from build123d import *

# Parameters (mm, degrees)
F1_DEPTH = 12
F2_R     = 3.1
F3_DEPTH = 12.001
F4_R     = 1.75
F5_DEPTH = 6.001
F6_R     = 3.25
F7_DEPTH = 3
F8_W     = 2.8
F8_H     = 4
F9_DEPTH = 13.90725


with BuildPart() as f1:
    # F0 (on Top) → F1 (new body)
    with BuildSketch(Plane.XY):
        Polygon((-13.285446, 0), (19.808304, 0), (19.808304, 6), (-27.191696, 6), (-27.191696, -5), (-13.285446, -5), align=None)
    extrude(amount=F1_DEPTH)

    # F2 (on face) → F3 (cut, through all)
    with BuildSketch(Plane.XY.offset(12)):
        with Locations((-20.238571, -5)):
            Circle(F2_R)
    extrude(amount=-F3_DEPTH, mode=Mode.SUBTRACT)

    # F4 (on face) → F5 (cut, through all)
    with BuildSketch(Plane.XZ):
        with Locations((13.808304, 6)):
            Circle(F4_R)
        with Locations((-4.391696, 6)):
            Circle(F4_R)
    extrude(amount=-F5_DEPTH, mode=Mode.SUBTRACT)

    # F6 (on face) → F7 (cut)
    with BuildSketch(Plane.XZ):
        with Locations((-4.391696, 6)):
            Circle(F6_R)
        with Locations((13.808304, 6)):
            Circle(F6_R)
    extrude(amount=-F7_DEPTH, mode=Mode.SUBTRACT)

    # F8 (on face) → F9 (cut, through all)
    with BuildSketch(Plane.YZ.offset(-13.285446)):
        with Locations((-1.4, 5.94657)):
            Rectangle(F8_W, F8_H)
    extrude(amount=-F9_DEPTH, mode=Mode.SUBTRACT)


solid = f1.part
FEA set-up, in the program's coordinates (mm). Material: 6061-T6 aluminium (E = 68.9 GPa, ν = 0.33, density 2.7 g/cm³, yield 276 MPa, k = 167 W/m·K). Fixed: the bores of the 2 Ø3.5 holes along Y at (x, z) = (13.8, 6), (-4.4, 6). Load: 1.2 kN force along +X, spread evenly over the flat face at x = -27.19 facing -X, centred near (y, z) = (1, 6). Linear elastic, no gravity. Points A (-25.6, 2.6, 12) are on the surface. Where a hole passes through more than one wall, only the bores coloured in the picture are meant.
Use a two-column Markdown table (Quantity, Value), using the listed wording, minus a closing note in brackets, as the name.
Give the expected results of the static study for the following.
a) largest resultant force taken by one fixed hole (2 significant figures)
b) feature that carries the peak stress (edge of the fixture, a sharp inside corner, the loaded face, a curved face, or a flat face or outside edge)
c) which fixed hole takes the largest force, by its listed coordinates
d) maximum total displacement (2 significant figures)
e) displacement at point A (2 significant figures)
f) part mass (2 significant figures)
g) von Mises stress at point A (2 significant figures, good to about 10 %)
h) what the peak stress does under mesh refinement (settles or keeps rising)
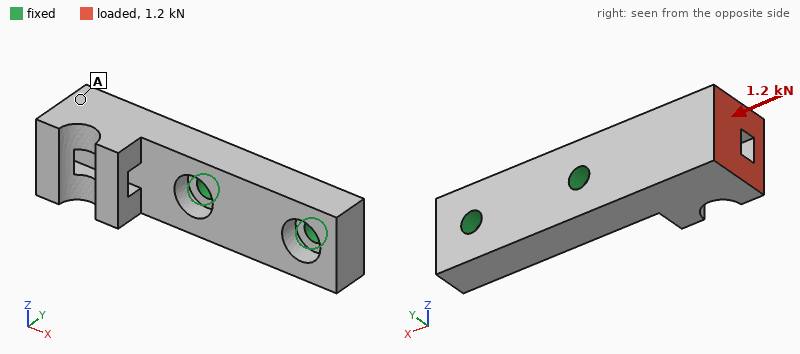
| Quantity | Value |
|---|---|
| largest resultant force taken by one fixed hole | 790 N |
| feature that carries the peak stress | edge of the fixture |
| which fixed hole takes the largest force, by its listed coordinates | (-4.4, 6) |
| maximum total displacement | 87 µm |
| displacement at point A | 68 µm |
| part mass | 9.8 g |
| von Mises stress at point A | 14 MPa |
| what the peak stress does under mesh refinement | keeps rising |
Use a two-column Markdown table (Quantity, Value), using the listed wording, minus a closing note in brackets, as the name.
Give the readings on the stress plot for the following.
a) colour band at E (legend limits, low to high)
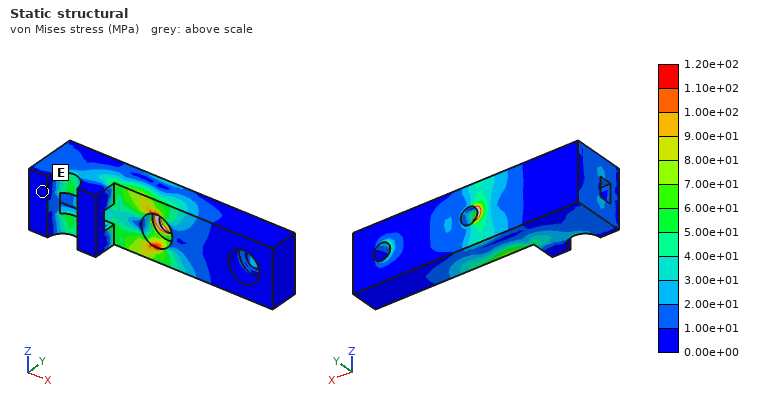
| Quantity | Value |
|---|---|
| colour band at E | 0.00e+00 to 1.00e+01 MPa |
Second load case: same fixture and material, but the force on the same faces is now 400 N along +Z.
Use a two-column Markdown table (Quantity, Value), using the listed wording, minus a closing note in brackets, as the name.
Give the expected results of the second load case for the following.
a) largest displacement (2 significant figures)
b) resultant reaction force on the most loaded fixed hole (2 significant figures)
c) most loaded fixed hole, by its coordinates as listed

| Quantity | Value |
|---|---|
| largest displacement | 67 µm |
| resultant reaction force on the most loaded fixed hole | 730 N |
| most loaded fixed hole, by its coordinates as listed | (-4.4, 6) |
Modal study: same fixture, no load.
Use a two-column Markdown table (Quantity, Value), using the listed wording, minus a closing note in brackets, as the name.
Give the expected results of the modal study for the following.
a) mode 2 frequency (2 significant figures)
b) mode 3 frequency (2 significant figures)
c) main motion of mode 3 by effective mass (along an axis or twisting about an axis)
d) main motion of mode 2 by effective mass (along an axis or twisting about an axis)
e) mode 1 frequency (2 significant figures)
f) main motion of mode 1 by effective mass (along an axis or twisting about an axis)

| Quantity | Value |
|---|---|
| mode 2 frequency | 9000 Hz |
| mode 3 frequency | 15 kHz |
| main motion of mode 3 by effective mass | twisting about X |
| main motion of mode 2 by effective mass | along Z |
| mode 1 frequency | 5600 Hz |
| main motion of mode 1 by effective mass | along Y |
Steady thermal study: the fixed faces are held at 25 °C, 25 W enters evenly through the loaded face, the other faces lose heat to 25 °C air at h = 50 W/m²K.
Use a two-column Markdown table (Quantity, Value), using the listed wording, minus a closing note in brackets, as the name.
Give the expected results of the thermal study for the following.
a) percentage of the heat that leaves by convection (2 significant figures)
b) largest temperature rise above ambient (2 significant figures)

| Quantity | Value |
|---|---|
| percentage of the heat that leaves by convection | 6.8 % |
| largest temperature rise above ambient | 46 K |
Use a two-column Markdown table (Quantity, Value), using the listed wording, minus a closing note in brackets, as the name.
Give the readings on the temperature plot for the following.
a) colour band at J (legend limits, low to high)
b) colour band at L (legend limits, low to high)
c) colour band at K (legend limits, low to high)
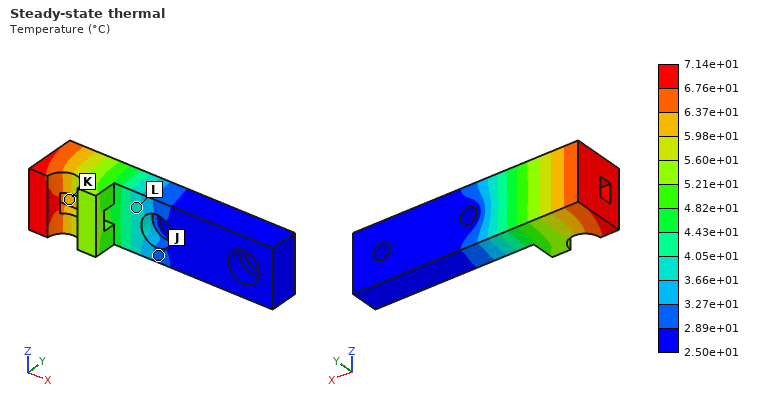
| Quantity | Value |
|---|---|
| colour band at J | 2.89e+01 to 3.27e+01 °C |
| colour band at L | 3.66e+01 to 4.05e+01 °C |
| colour band at K | 5.98e+01 to 6.37e+01 °C |
